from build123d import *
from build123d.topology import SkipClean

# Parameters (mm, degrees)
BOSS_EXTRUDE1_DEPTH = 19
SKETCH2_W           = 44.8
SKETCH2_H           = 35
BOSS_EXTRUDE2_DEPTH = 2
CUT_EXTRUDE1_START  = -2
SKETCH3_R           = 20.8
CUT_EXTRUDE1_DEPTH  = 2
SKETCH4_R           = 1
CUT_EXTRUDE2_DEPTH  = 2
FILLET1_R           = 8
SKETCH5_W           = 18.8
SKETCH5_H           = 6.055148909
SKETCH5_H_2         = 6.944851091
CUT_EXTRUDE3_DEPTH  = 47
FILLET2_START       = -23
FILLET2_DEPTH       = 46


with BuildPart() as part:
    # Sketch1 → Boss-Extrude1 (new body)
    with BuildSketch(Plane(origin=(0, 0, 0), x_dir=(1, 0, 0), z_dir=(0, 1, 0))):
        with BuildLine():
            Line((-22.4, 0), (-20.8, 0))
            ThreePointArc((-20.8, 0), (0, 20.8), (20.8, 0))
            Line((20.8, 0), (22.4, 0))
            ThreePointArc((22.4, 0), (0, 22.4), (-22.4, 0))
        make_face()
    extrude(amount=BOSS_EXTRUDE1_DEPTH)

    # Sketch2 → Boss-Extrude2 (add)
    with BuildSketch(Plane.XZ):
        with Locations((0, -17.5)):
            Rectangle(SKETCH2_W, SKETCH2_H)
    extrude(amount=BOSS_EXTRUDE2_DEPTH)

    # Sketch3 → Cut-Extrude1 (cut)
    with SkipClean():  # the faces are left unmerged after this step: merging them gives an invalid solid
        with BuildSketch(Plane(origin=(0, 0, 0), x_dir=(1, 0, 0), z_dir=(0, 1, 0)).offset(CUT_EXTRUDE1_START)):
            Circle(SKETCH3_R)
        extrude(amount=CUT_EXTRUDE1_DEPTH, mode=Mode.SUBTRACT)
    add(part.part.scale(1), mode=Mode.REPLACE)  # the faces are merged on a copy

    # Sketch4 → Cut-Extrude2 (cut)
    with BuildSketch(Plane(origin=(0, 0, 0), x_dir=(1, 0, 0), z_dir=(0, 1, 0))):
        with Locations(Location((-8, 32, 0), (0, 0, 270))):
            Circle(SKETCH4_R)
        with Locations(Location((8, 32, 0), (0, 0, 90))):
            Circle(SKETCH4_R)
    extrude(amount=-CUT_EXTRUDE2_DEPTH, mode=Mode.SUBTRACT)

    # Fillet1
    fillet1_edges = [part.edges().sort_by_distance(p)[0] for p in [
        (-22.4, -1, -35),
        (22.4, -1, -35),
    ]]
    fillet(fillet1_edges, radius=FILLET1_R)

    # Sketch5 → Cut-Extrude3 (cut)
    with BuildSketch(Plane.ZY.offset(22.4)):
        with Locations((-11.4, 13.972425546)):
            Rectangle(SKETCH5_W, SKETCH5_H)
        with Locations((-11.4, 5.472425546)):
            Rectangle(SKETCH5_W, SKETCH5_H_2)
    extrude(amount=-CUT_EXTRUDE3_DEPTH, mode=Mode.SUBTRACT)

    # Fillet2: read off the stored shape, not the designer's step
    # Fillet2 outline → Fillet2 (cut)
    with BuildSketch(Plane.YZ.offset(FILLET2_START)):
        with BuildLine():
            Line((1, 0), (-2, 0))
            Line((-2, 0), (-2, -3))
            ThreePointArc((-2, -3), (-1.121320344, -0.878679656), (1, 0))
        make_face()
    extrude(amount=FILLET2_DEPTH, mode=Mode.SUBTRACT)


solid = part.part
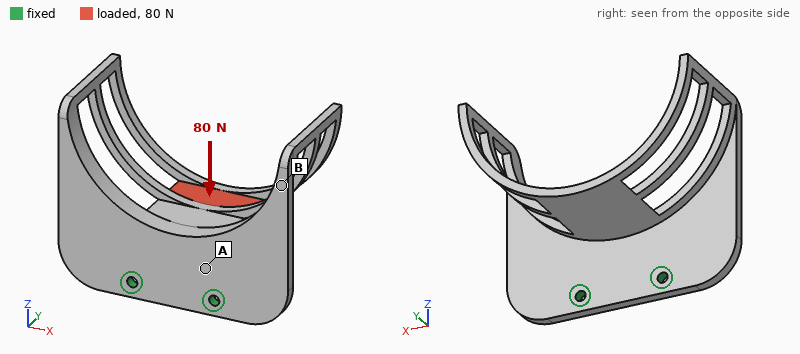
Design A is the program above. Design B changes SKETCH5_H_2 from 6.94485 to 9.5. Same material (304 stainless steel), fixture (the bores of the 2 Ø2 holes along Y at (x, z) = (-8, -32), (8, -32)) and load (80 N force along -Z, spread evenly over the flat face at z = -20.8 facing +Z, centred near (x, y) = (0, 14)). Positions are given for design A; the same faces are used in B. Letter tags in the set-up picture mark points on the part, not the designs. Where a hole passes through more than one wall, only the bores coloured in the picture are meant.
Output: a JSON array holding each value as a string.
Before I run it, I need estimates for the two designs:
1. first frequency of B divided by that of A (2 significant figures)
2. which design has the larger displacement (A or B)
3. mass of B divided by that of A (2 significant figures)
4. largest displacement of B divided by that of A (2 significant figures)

["1.0", "B", "0.92", "1.2"]
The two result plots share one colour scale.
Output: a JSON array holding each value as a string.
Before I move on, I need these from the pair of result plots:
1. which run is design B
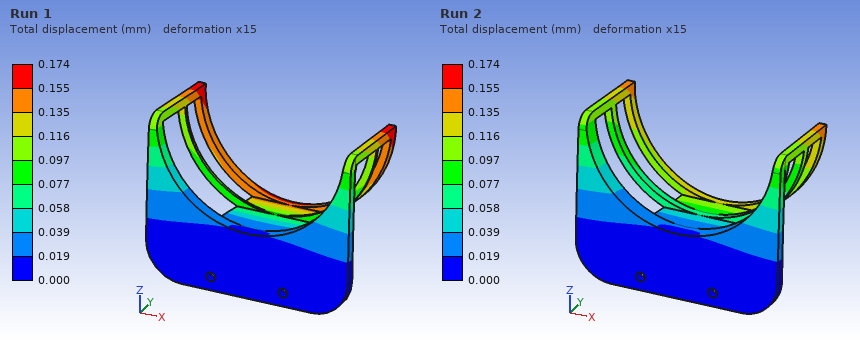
["Run 1"]
